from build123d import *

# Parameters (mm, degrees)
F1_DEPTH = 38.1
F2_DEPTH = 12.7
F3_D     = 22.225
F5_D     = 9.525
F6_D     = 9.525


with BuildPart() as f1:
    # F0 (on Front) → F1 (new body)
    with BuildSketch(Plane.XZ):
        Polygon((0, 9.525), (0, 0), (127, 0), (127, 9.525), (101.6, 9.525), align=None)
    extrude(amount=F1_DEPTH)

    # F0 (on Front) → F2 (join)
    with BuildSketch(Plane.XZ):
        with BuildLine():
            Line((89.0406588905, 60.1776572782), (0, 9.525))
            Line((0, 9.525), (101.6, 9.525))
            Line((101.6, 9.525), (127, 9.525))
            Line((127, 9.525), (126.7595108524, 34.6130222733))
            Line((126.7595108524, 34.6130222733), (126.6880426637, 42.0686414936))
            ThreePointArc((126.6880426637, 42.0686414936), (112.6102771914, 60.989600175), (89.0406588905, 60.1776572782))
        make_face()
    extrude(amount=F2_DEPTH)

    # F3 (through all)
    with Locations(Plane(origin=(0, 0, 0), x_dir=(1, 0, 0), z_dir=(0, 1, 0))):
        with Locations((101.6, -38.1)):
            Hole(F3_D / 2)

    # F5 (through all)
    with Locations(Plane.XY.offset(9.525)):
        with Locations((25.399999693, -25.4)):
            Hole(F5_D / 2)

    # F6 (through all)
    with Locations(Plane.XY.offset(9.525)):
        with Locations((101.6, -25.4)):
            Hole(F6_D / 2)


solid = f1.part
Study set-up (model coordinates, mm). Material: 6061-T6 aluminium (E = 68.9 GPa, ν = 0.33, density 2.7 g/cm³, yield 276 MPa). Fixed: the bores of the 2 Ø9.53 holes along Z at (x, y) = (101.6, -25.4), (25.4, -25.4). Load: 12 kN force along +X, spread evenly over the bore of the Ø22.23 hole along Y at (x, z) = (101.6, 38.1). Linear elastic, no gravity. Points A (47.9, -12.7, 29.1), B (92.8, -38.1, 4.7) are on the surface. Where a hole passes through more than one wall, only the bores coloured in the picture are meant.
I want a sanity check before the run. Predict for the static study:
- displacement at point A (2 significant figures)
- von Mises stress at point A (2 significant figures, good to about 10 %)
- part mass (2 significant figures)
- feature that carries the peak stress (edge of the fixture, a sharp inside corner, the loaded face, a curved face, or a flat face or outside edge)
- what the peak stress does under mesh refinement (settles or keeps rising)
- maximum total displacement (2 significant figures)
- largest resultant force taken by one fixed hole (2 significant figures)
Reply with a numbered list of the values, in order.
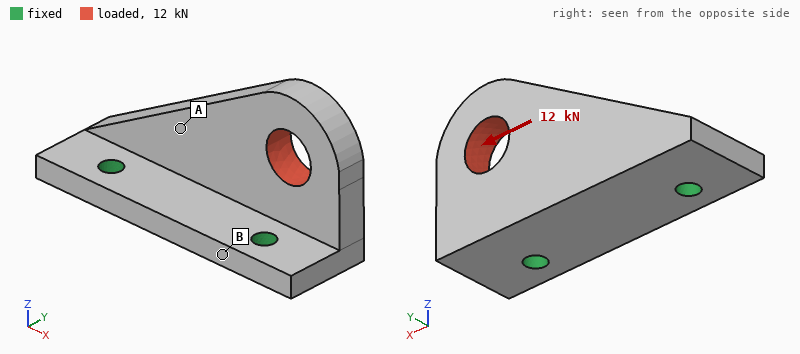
1. 0.048 mm
2. 45 MPa
3. 250 g
4. edge of the fixture
5. keeps rising
6. 0.14 mm
7. 8.3 kN
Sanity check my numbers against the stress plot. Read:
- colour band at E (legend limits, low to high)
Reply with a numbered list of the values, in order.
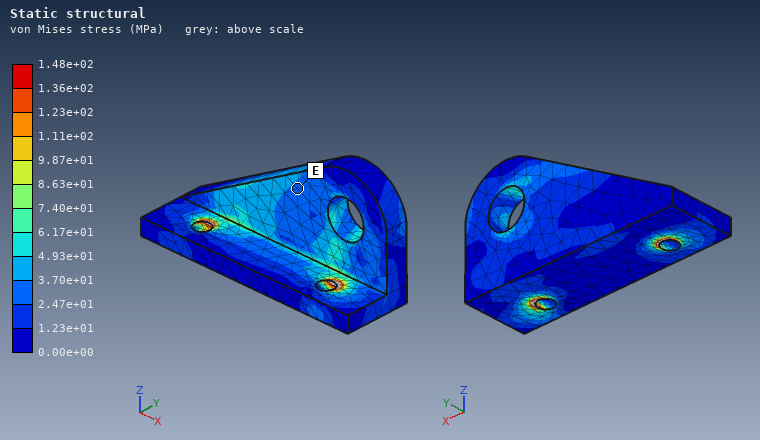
1. 2.47e+01 to 3.70e+01 MPa
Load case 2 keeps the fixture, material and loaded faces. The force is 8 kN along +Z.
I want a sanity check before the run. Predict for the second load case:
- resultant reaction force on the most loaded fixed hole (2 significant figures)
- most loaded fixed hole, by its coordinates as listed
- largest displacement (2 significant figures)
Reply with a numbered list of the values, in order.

1. 7.7 kN
2. (101.6, -25.4)
3. 0.26 mm
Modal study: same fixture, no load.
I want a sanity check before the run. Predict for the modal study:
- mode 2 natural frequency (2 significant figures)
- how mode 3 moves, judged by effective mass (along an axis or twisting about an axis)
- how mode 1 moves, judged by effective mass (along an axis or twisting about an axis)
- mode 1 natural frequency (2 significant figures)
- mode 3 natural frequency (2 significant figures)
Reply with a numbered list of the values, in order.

1. 4900 Hz
2. along Z
3. along Y
4. 2100 Hz
5. 6200 Hz
